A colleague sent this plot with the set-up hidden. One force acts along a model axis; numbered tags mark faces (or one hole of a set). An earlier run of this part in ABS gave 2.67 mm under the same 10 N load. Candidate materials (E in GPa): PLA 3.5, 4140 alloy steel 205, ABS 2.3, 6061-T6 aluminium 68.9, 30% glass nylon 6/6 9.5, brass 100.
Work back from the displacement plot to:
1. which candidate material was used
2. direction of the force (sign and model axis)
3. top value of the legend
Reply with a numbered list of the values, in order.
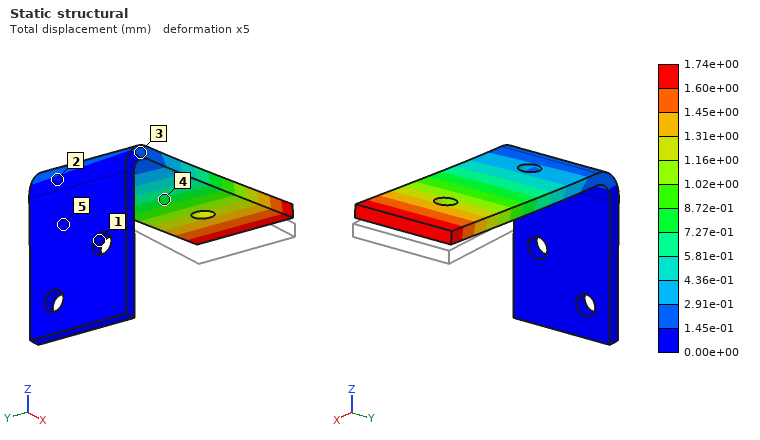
1. PLA
2. +Z
3. 1.74e+00 mm
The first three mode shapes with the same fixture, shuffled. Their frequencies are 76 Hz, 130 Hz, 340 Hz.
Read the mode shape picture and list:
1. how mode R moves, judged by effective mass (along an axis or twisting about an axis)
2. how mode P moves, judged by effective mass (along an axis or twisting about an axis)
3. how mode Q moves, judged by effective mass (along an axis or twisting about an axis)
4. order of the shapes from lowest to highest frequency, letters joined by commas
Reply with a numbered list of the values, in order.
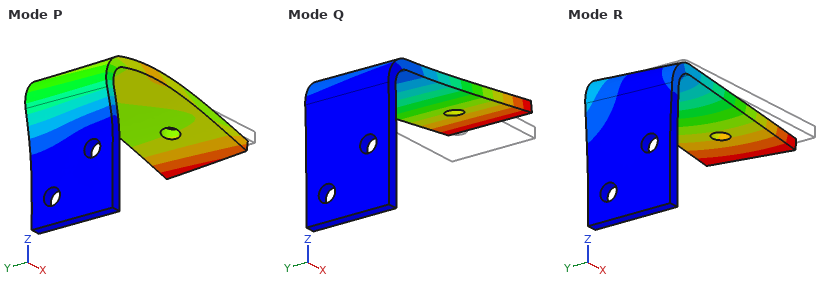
1. along Y
2. along X
3. along Z
4. Q, R, P
